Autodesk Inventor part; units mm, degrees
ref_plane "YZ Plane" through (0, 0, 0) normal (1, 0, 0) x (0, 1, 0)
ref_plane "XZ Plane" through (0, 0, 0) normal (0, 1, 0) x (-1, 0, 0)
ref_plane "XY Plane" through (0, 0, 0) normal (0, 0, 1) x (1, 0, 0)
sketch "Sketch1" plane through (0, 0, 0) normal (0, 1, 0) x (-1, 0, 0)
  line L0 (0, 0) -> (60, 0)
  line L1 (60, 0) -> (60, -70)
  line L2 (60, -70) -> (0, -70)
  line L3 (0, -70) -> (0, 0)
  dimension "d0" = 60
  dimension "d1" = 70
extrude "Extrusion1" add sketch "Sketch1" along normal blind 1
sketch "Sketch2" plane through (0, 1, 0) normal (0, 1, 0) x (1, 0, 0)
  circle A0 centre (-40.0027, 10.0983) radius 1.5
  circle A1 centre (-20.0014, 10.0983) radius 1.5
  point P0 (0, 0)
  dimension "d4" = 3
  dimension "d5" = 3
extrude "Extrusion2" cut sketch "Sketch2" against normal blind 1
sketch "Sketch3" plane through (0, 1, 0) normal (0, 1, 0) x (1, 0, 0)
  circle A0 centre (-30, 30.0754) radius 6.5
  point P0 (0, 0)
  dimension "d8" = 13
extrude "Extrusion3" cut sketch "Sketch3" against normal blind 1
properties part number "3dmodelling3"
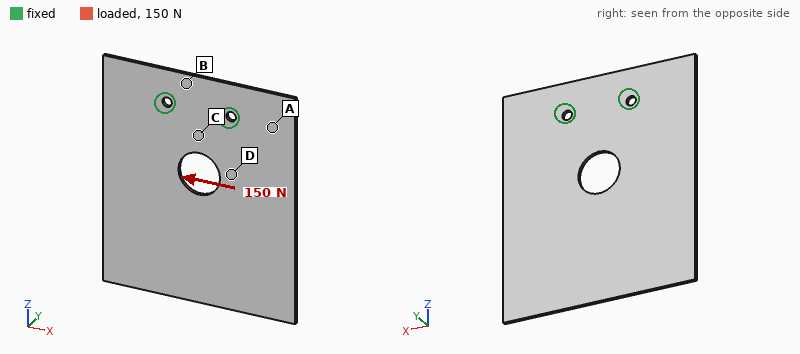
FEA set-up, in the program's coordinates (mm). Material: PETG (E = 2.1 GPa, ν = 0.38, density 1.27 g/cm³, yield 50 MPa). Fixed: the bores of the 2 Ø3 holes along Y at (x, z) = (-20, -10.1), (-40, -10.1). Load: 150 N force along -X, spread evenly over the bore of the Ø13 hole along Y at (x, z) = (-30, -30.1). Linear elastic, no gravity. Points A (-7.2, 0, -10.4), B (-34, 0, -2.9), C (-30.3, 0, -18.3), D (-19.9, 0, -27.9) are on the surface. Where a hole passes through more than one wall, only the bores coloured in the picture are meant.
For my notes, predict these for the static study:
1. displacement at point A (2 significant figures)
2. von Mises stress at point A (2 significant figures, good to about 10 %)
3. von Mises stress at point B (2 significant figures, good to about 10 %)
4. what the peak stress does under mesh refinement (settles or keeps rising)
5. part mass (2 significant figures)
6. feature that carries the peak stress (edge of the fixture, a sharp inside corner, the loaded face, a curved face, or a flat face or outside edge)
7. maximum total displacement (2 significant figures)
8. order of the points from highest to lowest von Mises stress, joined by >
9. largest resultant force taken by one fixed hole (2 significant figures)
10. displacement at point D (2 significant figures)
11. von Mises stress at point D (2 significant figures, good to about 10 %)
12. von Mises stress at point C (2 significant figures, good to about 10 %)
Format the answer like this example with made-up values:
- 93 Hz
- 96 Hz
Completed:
- 0.15 mm
- 2.0 MPa
- 3.9 MPa
- keeps rising
- 5.1 g
- edge of the fixture
- 0.56 mm
- C > D > B > A
- 150 N
- 0.21 mm
- 6.7 MPa
- 14 MPa
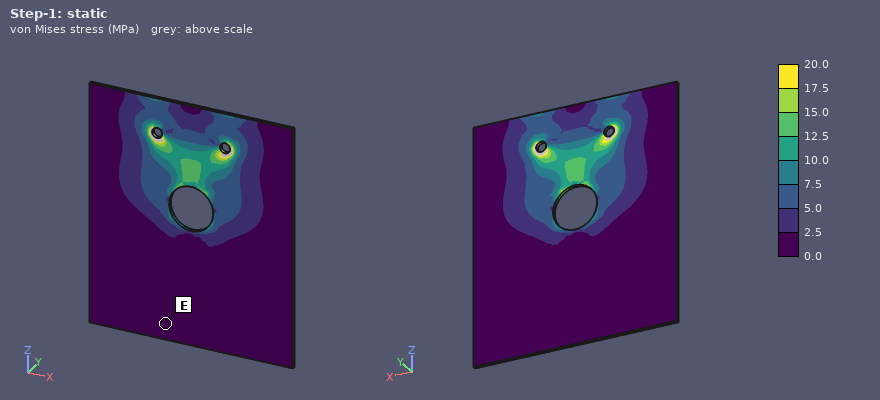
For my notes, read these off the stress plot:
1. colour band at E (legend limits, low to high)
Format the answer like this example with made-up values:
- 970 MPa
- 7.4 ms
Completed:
- 0.0 to 2.5 MPa
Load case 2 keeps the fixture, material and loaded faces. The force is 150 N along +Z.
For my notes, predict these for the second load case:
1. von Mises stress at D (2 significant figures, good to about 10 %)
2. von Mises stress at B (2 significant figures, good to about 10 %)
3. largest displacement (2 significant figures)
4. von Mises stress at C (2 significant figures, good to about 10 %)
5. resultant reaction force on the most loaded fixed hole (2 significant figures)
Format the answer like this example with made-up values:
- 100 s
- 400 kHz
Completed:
- 3.7 MPa
- 1.3 MPa
- 74 µm
- 3.1 MPa
- 76 N
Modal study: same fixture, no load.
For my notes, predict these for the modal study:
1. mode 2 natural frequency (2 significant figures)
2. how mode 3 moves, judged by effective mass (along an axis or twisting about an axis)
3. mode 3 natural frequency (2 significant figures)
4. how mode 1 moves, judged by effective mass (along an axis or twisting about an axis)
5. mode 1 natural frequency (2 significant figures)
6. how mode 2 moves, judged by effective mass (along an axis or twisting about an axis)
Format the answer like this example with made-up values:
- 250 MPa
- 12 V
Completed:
- 120 Hz
- along Y
- 310 Hz
- along Y
- 54 Hz
- twisting about Z
